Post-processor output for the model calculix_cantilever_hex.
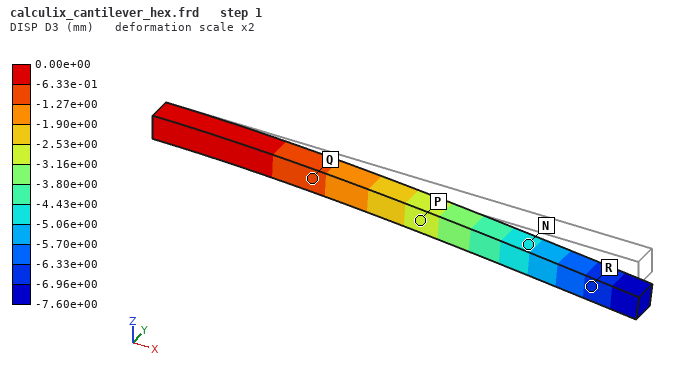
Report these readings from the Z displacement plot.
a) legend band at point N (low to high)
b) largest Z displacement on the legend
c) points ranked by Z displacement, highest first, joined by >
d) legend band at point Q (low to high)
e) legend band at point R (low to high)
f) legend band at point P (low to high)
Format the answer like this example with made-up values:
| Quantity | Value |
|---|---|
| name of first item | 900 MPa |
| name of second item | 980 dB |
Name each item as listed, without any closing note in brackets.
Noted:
| Quantity | Value |
|---|---|
| legend band at point N | -5.06e+00 to -4.43e+00 mm |
| largest Z displacement on the legend | 0.00e+00 mm |
| points ranked by Z displacement, highest first, joined by > | Q > P > N > R |
| legend band at point Q | -1.27e+00 to -6.33e-01 mm |
| legend band at point R | -6.96e+00 to -6.33e+00 mm |
| legend band at point P | -3.16e+00 to -2.53e+00 mm |
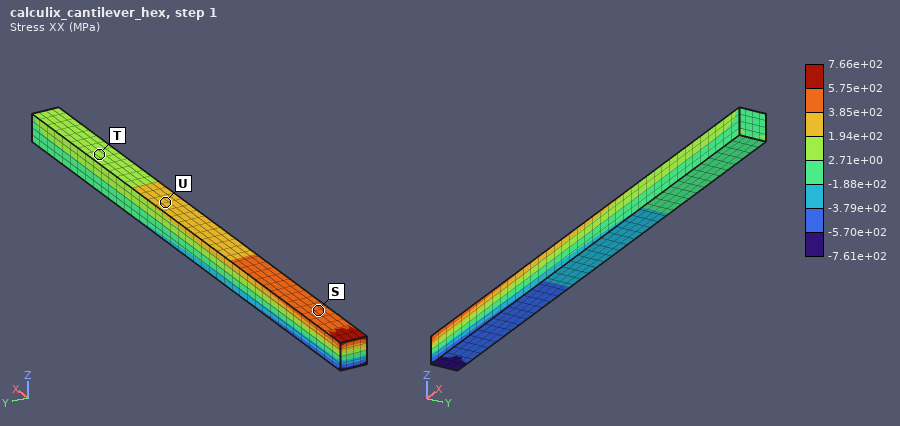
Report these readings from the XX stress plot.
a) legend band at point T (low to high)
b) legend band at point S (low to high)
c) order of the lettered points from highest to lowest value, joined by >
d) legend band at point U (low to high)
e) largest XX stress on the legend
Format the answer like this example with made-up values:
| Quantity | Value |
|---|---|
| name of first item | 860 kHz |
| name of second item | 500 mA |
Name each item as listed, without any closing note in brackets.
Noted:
| Quantity | Value |
|---|---|
| legend band at point T | 2.71e+00 to 1.94e+02 MPa |
| legend band at point S | 3.85e+02 to 5.75e+02 MPa |
| order of the lettered points from highest to lowest value, joined by > | S > U > T |
| legend band at point U | 1.94e+02 to 3.85e+02 MPa |
| largest XX stress on the legend | 7.66e+02 MPa |
